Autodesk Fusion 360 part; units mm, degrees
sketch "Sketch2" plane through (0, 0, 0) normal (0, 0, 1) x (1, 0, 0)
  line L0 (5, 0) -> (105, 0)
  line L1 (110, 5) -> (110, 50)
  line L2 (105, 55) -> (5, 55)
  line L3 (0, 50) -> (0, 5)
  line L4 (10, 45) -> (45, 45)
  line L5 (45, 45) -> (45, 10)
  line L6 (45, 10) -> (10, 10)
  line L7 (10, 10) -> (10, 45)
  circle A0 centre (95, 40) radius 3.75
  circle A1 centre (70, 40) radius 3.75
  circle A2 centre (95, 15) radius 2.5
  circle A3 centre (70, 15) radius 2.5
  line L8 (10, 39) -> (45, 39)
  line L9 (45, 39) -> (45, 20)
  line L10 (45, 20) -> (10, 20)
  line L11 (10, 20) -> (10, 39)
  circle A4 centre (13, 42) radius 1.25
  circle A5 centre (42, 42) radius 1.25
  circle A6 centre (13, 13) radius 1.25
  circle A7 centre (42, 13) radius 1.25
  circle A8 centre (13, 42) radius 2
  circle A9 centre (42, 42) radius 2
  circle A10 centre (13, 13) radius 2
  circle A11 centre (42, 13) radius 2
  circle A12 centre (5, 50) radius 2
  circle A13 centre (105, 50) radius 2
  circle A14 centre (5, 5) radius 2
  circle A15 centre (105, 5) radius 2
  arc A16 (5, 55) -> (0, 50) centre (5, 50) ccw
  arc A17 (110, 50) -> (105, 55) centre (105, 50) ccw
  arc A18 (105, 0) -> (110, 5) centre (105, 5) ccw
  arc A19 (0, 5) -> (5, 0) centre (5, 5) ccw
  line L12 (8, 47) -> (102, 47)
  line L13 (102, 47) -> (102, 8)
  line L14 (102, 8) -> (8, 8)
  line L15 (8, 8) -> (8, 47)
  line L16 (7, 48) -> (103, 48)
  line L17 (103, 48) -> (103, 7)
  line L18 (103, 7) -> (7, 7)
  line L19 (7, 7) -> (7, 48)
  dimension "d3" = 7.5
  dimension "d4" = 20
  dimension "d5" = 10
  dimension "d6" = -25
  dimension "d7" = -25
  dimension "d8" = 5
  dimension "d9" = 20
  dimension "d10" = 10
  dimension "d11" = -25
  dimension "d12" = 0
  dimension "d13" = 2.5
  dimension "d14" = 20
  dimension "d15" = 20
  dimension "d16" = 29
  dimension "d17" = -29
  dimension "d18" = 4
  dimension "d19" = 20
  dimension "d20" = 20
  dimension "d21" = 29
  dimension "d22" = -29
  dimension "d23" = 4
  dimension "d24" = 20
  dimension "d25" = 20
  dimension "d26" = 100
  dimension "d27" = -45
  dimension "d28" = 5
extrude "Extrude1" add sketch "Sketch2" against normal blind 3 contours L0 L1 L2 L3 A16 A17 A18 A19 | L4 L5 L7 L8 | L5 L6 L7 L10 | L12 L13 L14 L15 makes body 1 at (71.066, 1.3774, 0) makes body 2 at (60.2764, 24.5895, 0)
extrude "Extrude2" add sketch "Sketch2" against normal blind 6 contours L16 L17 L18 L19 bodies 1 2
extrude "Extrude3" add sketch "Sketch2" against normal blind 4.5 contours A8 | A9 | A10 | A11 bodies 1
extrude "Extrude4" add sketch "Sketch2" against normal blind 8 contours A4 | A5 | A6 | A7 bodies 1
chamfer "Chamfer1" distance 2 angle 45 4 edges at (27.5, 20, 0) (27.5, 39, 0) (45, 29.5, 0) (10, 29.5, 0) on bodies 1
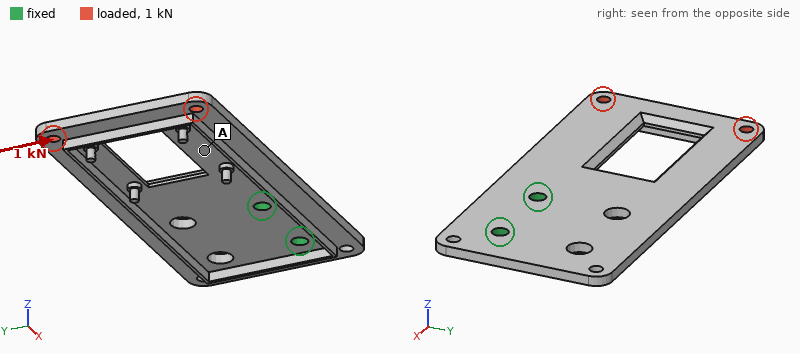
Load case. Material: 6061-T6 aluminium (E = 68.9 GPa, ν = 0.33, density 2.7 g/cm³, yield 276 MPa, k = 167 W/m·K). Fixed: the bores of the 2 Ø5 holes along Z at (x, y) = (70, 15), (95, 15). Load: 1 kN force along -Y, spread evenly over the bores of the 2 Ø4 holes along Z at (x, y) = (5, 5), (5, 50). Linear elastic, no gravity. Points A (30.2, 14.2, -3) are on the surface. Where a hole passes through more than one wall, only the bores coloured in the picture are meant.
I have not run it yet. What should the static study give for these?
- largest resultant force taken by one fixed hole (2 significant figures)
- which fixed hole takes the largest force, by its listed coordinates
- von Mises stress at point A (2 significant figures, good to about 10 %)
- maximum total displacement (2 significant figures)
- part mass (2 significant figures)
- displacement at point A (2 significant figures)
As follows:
3.2 kN
(70, 15)
24 MPa
0.25 mm
44 g
0.11 mm
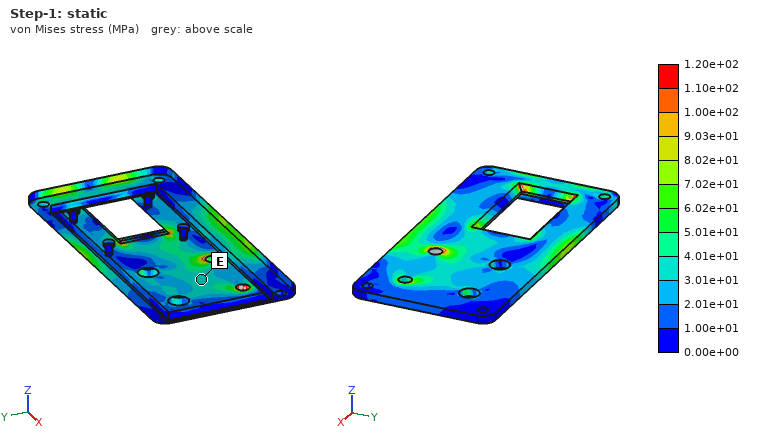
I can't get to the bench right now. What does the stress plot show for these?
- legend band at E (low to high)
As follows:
3.01e+01 to 4.01e+01 MPa
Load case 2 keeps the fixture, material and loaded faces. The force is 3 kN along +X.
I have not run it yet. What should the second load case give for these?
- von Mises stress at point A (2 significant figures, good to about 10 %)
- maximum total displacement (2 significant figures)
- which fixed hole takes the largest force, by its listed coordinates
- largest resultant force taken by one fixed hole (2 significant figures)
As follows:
18 MPa
0.14 mm
(70, 15)
2.4 kN
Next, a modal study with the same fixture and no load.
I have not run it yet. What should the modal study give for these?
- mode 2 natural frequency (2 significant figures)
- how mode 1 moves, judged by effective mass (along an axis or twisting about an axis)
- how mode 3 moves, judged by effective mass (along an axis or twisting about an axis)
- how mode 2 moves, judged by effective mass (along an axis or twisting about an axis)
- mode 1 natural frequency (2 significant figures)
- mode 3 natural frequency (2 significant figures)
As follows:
1000 Hz
along Z
along Z
twisting about X
540 Hz
1900 Hz
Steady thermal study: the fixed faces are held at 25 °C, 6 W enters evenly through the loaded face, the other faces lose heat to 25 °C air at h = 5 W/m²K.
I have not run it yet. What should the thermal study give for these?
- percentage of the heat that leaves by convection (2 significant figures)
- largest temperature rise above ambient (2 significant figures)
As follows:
8.2 %
23 K
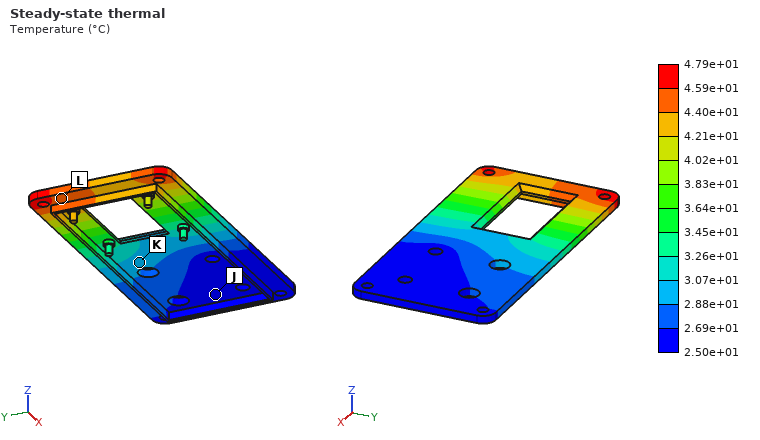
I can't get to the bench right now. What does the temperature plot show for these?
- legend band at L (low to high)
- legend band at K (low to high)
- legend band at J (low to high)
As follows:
4.40e+01 to 4.59e+01 °C
2.88e+01 to 3.07e+01 °C
2.50e+01 to 2.69e+01 °C
